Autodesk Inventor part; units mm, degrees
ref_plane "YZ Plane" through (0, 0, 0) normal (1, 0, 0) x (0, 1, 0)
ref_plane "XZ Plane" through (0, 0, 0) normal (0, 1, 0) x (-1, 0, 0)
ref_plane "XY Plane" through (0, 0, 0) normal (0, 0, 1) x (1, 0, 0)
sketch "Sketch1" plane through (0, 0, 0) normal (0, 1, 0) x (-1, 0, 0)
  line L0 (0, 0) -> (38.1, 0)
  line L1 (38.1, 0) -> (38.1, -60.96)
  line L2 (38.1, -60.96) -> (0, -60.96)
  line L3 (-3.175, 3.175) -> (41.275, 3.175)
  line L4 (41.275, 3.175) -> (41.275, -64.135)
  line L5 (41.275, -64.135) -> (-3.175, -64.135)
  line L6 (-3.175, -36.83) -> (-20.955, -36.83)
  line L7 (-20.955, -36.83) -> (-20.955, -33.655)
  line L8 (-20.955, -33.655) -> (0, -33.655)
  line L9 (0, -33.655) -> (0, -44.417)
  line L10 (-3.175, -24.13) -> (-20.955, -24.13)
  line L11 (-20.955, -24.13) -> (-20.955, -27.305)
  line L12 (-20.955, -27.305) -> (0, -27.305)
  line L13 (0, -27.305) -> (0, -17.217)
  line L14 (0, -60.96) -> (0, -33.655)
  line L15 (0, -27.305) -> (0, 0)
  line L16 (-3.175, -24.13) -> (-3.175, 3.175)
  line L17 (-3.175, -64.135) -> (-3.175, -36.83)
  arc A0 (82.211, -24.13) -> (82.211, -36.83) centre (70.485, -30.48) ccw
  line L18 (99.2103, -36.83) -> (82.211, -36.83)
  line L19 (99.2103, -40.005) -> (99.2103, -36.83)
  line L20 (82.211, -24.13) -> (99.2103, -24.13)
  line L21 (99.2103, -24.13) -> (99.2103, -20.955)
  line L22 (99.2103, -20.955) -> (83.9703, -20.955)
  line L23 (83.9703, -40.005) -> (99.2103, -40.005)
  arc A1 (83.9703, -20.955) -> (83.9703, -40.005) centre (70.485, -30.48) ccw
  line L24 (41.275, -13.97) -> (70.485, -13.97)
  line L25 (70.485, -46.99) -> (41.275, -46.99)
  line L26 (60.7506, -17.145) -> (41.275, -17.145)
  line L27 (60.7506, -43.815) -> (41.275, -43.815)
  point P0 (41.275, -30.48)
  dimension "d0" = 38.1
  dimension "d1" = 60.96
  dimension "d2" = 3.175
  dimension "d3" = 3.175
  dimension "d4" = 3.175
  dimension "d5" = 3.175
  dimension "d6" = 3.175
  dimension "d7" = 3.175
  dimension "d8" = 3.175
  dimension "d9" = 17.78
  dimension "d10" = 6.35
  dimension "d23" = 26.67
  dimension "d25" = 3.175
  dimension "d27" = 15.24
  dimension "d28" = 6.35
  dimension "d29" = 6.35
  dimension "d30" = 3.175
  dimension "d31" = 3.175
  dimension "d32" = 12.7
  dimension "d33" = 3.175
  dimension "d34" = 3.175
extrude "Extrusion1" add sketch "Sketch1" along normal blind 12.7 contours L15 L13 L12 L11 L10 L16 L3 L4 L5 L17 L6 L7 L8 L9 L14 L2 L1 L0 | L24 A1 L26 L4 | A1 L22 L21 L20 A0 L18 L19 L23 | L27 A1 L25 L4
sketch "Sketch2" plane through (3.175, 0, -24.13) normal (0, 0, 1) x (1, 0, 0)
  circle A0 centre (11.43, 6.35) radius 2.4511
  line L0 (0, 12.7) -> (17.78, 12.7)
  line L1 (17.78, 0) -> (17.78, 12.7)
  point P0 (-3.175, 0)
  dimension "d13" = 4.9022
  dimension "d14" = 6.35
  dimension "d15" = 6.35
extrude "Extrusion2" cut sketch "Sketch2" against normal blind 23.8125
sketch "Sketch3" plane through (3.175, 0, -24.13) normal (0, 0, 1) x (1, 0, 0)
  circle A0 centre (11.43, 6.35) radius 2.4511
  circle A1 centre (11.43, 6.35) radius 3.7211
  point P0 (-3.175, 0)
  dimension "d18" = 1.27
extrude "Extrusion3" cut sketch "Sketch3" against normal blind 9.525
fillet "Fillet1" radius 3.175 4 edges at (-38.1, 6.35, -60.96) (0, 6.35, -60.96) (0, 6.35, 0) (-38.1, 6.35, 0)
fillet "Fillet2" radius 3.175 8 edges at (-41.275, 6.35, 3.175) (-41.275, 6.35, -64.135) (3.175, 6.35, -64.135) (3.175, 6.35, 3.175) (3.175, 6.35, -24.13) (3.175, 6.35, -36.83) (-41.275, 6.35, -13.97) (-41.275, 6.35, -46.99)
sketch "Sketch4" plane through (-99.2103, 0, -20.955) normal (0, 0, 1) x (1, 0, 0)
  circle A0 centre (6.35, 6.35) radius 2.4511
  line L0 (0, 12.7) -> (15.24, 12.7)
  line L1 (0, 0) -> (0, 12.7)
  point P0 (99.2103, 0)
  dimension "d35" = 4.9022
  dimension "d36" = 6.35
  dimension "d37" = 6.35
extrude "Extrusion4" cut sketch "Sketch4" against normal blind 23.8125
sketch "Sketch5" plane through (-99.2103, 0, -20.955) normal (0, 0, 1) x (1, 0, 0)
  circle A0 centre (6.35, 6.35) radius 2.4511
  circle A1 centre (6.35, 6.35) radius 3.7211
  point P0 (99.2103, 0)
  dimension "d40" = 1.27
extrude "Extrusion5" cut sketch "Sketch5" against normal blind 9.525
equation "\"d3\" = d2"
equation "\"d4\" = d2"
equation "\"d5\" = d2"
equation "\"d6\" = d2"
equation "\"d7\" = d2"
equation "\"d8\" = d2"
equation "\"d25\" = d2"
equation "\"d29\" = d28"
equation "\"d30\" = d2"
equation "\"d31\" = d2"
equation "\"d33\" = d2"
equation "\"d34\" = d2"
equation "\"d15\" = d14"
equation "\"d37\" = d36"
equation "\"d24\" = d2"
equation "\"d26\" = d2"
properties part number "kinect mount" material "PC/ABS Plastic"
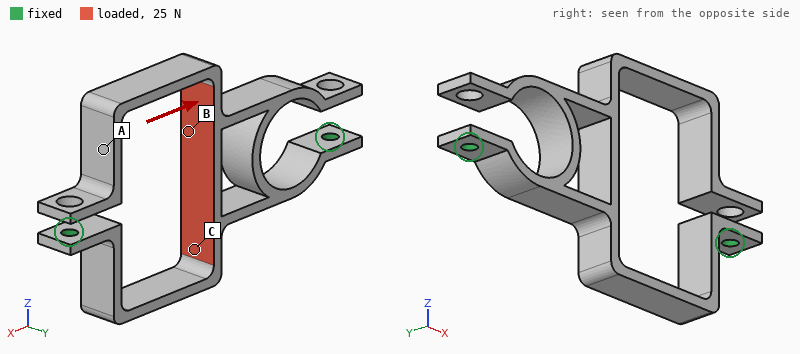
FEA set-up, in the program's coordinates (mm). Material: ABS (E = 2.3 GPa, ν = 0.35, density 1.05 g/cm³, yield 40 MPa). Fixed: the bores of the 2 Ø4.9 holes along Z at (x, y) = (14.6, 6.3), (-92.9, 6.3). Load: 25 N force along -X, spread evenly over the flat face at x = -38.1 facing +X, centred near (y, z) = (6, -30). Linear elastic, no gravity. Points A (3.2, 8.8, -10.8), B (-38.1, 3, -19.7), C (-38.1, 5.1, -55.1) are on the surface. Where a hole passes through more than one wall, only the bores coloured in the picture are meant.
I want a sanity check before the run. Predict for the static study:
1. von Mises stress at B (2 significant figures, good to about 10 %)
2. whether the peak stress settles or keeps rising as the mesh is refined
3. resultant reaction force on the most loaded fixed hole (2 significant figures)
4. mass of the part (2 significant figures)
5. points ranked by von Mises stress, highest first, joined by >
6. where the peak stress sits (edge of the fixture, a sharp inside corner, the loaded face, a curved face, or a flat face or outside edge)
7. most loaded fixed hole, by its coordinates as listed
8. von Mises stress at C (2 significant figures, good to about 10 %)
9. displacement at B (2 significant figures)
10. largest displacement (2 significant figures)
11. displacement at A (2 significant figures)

1.6 MPa
keeps rising
29 N
16 g
C > B > A
edge of the fixture
(-92.9, 6.3)
4.4 MPa
0.73 mm
1.6 mm
1.4 mm
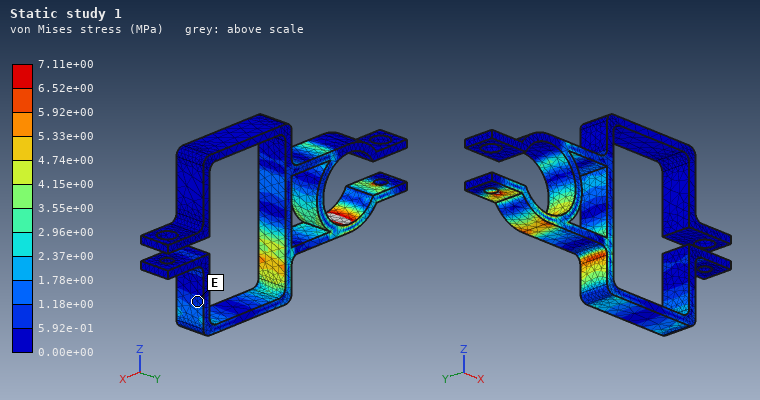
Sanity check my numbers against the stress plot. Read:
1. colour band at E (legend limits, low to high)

5.92e-01 to 1.18e+00 MPa
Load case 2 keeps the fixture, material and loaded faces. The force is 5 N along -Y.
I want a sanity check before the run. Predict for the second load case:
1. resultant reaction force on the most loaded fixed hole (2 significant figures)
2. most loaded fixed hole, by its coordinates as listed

3.7 N
(-92.9, 6.3)
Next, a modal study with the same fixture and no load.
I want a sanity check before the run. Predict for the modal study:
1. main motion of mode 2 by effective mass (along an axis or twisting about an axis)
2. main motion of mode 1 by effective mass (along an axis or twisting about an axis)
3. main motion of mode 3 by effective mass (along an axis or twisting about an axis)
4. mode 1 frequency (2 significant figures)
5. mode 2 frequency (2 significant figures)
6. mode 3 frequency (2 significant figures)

along Z
along Y
along X
84 Hz
95 Hz
180 Hz
